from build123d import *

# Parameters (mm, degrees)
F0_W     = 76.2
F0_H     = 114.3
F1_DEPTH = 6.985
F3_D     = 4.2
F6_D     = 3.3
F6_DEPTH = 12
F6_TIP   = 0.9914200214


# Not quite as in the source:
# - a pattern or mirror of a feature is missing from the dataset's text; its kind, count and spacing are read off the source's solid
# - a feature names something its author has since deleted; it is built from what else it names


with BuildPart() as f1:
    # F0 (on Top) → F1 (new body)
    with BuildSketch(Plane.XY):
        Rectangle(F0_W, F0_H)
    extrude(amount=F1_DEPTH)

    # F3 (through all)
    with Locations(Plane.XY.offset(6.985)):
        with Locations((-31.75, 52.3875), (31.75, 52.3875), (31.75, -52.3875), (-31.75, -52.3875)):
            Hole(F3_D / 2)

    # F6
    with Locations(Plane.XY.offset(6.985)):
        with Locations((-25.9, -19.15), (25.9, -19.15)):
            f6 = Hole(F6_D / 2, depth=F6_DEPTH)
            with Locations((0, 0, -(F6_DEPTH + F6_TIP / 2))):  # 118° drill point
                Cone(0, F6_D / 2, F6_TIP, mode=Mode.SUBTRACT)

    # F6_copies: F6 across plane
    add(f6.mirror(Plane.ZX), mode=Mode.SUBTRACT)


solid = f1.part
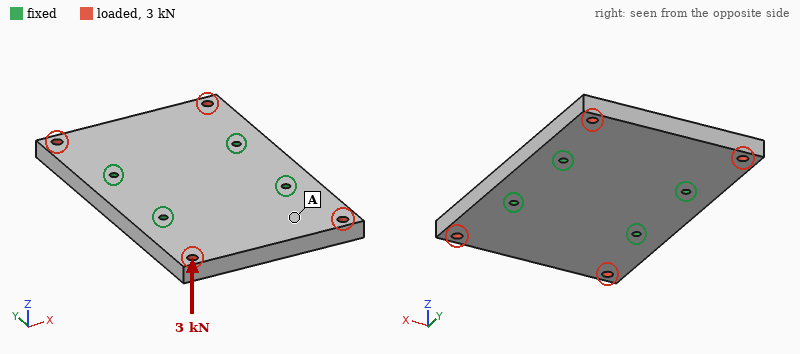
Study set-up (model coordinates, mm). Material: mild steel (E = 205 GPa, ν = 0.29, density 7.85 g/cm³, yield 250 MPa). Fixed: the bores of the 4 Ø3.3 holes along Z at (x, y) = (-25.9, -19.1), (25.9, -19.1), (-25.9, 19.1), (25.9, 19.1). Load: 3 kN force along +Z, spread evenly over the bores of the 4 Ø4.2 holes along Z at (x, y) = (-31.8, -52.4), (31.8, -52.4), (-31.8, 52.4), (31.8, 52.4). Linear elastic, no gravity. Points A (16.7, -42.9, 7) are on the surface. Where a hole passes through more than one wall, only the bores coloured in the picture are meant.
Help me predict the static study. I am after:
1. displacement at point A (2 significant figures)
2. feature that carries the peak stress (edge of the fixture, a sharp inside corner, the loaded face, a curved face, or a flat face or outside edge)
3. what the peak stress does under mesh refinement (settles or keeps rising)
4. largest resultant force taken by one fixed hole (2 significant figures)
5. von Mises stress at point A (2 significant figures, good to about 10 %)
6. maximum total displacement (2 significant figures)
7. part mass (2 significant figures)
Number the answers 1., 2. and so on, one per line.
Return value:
1. 36 µm
2. edge of the fixture
3. keeps rising
4. 750 N
5. 28 MPa
6. 78 µm
7. 470 g
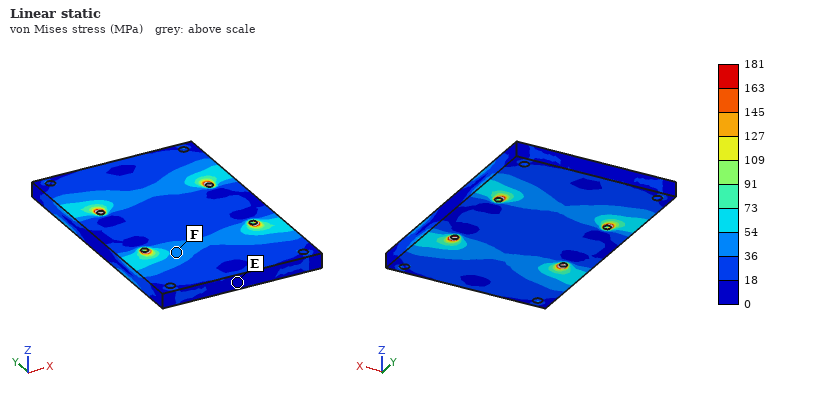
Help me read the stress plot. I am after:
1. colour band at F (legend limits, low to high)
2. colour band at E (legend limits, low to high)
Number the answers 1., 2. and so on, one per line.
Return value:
1. 36 to 54 MPa
2. 0 to 18 MPa
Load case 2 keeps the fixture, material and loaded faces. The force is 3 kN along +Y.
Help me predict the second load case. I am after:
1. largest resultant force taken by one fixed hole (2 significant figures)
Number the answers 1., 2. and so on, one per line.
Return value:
1. 750 N
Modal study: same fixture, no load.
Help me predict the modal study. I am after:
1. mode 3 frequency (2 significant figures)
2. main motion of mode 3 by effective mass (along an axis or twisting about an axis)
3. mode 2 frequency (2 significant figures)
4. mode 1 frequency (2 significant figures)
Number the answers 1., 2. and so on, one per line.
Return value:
1. 5600 Hz
2. twisting about Y
3. 3300 Hz
4. 3200 Hz
